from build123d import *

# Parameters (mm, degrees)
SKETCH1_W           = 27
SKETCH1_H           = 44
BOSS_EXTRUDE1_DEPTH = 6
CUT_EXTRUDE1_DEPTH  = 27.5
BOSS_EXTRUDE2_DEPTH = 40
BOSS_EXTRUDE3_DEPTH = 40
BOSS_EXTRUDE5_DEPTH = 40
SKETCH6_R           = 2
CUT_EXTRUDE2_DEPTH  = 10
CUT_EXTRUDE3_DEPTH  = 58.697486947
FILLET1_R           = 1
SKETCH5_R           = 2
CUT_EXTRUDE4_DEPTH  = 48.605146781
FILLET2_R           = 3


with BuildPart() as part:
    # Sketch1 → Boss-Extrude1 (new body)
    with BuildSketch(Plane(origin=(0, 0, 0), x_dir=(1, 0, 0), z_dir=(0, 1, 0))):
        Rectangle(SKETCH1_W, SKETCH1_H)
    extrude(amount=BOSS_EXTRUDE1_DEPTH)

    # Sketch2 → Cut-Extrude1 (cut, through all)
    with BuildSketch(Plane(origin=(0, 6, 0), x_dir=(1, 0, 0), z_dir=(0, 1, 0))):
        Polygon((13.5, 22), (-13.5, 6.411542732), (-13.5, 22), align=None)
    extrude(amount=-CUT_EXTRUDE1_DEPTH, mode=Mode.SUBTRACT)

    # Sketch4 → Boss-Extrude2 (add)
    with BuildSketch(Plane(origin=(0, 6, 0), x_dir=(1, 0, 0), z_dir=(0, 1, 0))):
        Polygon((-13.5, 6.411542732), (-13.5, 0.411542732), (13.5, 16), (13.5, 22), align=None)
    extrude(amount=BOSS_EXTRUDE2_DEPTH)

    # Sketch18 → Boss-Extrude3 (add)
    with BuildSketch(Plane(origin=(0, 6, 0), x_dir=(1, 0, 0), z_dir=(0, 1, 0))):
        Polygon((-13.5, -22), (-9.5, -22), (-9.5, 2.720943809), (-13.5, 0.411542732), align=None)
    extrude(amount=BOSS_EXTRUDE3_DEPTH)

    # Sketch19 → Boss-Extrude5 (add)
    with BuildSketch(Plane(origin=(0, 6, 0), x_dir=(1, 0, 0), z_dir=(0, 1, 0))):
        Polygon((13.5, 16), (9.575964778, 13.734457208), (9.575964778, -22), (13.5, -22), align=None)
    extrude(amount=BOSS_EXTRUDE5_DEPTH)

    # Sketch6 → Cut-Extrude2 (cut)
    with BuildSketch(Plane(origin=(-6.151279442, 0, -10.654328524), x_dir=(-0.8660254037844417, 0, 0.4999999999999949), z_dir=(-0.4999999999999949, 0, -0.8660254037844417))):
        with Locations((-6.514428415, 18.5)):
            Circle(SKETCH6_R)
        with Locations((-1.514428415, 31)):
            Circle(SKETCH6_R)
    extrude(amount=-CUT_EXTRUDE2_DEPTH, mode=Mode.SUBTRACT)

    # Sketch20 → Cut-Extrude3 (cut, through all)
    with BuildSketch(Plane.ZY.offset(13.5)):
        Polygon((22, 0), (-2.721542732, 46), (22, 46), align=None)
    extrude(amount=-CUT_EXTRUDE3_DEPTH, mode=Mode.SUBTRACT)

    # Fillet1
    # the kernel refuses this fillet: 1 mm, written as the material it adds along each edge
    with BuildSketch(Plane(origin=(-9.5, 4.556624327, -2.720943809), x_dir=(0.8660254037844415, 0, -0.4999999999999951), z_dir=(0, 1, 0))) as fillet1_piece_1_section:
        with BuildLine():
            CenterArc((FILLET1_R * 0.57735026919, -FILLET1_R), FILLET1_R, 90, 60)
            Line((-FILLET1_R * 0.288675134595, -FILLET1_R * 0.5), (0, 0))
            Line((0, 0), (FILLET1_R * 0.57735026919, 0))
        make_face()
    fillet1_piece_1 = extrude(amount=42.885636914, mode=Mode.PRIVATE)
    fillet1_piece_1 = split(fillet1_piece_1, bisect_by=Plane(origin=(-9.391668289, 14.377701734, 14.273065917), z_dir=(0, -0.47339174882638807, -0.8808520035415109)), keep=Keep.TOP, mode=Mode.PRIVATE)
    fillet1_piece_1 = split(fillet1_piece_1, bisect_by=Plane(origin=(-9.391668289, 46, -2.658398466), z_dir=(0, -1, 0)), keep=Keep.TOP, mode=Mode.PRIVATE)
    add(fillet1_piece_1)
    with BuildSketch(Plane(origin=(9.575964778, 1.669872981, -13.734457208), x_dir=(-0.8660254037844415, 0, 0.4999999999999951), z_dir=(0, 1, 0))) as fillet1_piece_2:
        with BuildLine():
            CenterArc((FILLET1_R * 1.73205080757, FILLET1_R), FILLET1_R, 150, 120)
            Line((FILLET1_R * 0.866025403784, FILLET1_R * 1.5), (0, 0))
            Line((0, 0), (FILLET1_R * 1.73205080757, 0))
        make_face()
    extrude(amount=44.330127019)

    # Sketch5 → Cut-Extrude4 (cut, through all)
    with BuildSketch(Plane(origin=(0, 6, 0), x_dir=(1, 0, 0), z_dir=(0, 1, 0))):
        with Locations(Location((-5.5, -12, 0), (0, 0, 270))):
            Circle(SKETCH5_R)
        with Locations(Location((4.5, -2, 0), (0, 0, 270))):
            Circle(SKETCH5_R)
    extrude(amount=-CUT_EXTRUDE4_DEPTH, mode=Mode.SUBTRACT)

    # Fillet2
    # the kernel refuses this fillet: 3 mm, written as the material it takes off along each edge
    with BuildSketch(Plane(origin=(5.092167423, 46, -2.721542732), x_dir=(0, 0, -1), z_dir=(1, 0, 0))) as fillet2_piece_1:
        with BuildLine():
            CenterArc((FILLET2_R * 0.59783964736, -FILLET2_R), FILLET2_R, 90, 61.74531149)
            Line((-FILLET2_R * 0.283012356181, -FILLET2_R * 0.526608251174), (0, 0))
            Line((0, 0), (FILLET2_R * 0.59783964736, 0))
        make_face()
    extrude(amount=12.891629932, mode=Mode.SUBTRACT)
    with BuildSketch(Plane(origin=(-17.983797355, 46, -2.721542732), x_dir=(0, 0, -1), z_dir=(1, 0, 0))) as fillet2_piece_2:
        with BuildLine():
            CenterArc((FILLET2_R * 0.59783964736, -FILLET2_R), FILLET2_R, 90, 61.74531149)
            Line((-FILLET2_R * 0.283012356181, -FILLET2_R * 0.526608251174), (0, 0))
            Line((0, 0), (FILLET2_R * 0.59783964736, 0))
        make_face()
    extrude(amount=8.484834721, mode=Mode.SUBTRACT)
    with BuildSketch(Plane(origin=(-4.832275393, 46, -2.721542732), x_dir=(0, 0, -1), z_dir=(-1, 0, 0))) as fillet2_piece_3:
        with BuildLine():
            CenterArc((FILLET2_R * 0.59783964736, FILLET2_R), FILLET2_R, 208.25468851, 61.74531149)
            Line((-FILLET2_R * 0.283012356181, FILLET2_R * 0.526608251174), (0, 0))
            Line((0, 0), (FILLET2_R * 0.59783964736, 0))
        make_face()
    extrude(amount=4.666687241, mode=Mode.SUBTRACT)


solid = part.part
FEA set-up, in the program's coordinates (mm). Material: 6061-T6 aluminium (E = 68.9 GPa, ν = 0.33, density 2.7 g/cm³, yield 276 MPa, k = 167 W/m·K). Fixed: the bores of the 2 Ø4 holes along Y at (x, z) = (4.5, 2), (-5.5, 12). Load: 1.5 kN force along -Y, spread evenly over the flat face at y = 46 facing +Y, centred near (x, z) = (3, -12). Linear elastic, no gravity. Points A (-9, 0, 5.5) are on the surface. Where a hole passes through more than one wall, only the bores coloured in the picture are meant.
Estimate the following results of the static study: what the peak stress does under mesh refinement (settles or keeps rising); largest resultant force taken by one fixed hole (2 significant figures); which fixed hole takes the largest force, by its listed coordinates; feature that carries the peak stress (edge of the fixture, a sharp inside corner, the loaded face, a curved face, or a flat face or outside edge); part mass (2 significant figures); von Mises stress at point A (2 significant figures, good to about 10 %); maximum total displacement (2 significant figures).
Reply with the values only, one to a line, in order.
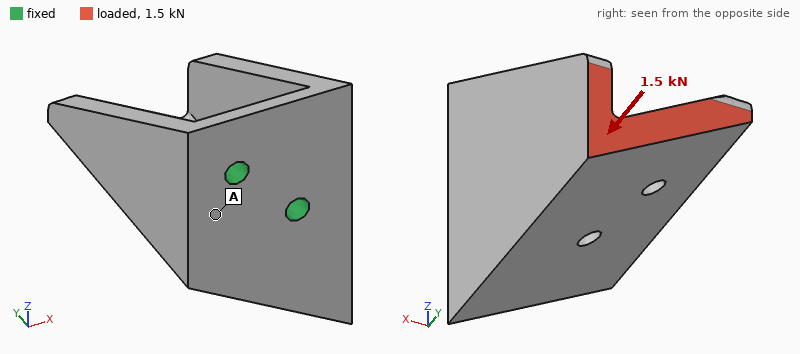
keeps rising
1.8 kN
(4.5, 2)
edge of the fixture
46 g
23 MPa
93 µm
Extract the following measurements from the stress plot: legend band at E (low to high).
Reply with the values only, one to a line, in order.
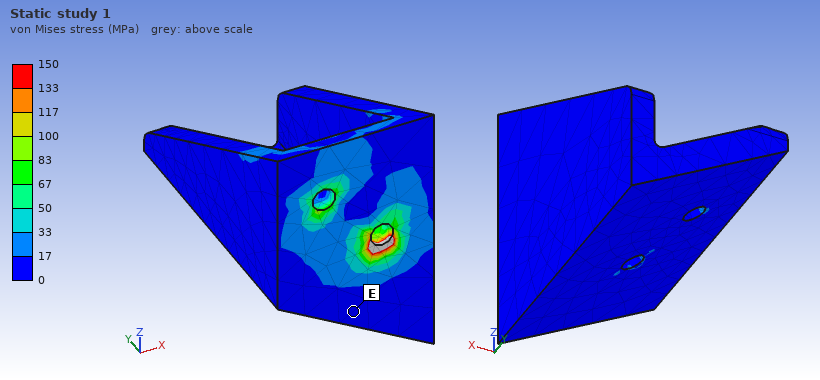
0 to 17 MPa
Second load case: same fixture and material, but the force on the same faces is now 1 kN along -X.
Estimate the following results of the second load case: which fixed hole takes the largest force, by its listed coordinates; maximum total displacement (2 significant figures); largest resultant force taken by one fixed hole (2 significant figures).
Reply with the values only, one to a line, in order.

(4.5, 2)
0.29 mm
2.0 kN
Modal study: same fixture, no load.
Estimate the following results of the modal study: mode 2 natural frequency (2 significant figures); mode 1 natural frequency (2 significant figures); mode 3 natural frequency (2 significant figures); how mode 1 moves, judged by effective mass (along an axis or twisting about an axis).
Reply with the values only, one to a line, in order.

3900 Hz
3100 Hz
9400 Hz
along X
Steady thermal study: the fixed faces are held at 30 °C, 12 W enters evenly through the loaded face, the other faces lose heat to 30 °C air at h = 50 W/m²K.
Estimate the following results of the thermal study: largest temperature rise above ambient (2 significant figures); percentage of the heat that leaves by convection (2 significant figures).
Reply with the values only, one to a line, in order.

14 K
16 %
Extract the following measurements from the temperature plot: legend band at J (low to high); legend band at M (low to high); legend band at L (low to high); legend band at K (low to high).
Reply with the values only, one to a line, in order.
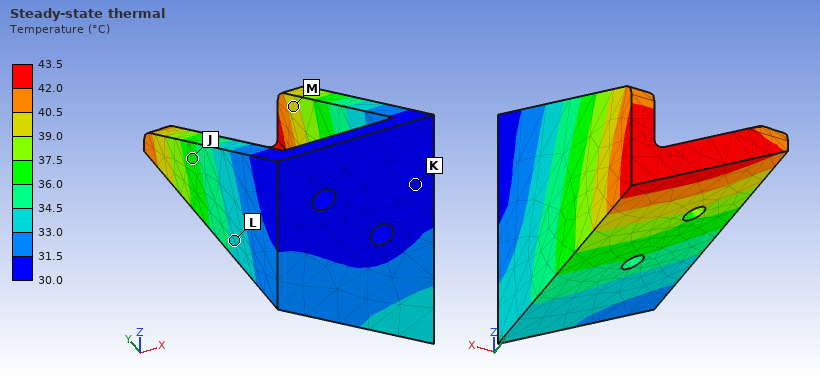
36.0 to 37.5 °C
39.0 to 40.5 °C
33.0 to 34.5 °C
30.0 to 31.5 °C
